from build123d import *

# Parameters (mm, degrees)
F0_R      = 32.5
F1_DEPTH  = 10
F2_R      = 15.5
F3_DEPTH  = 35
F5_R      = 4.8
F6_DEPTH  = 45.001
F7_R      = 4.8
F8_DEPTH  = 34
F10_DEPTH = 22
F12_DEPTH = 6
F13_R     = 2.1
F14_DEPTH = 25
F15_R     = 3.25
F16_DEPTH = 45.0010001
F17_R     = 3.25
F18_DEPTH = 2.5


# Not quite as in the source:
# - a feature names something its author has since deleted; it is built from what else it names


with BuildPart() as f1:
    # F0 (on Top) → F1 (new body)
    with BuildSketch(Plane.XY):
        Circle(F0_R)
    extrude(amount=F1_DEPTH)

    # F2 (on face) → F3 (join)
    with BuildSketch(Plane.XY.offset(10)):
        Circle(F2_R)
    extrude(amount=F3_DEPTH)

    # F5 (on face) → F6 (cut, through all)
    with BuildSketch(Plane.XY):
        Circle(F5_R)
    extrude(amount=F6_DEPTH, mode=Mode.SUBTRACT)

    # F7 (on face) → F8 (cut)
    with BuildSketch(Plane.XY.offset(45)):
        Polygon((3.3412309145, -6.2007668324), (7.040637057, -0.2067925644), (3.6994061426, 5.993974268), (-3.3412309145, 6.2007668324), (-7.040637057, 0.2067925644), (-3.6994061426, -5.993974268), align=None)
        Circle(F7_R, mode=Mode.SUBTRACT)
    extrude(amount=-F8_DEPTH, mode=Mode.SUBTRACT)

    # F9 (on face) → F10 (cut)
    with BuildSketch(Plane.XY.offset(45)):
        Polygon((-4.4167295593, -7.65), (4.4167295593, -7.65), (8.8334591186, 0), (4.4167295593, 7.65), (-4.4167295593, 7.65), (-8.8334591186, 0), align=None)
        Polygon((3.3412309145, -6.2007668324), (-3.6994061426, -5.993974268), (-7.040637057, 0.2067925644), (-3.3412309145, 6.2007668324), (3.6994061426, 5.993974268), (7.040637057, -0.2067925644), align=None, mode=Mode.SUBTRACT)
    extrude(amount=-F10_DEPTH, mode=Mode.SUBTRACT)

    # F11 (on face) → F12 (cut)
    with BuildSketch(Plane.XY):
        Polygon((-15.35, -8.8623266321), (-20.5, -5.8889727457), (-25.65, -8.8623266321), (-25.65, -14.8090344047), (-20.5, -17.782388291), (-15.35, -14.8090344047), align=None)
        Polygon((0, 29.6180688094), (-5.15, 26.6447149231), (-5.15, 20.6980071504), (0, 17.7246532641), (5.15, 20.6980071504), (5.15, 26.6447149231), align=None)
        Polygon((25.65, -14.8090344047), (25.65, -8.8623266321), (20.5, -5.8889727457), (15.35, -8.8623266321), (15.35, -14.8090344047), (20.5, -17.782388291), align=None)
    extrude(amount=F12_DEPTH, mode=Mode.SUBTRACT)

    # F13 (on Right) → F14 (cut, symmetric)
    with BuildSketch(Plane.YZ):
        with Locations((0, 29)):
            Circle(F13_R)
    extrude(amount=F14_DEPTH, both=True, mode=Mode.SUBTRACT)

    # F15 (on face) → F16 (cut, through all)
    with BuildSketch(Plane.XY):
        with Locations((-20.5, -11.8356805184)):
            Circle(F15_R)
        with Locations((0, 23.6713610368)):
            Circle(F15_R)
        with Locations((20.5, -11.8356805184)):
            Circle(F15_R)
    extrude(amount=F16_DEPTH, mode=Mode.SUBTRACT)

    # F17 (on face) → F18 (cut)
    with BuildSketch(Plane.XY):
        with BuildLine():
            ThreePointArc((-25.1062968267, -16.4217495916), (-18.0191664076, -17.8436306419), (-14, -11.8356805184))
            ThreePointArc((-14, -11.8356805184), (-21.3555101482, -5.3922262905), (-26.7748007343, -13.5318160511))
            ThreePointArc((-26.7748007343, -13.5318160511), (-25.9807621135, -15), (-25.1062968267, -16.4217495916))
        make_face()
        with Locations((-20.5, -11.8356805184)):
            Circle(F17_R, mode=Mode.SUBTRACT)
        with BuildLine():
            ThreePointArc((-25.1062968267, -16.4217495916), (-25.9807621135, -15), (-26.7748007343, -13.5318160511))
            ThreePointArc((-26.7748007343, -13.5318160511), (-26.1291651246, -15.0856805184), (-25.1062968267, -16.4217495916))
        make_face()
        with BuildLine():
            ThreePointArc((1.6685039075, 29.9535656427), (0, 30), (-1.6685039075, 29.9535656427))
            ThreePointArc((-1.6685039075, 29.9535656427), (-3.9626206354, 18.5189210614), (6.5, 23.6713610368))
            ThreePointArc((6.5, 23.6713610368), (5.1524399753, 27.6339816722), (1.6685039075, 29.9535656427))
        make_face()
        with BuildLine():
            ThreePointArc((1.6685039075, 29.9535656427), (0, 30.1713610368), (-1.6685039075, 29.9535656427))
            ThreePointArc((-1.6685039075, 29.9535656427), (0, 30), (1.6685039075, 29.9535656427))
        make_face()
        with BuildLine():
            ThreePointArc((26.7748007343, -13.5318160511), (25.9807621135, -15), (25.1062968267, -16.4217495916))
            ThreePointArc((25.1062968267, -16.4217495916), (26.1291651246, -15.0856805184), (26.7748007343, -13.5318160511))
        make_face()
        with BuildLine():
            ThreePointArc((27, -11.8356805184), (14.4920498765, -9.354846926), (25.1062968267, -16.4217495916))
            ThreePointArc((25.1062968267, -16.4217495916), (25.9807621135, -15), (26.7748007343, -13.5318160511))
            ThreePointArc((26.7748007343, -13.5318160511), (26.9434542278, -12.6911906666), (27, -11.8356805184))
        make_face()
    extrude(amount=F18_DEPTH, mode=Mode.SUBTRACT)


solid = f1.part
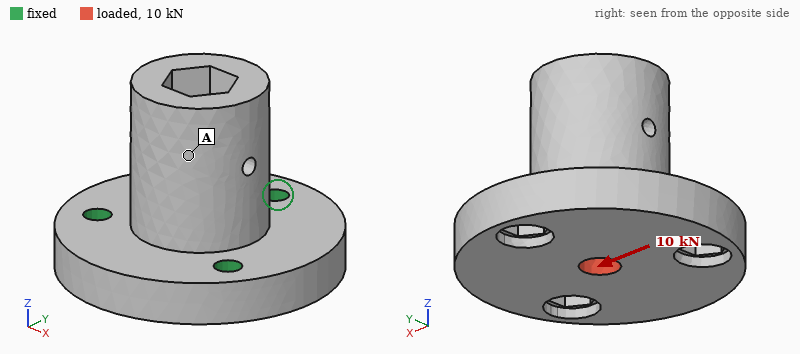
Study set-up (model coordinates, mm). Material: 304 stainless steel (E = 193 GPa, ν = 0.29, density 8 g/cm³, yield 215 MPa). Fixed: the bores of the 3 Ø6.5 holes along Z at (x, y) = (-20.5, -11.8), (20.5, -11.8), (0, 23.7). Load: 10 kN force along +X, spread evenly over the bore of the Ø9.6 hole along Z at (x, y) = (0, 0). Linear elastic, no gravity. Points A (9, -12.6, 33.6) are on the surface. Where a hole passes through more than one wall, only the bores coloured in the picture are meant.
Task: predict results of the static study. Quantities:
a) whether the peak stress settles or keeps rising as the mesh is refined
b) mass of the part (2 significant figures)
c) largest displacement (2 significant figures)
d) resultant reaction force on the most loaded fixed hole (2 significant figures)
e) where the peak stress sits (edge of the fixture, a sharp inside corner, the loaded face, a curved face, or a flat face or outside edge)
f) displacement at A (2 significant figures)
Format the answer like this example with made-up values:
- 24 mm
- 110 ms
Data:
- keeps rising
- 400 g
- 4.4 µm
- 3.6 kN
- edge of the fixture
- 1.6 µm
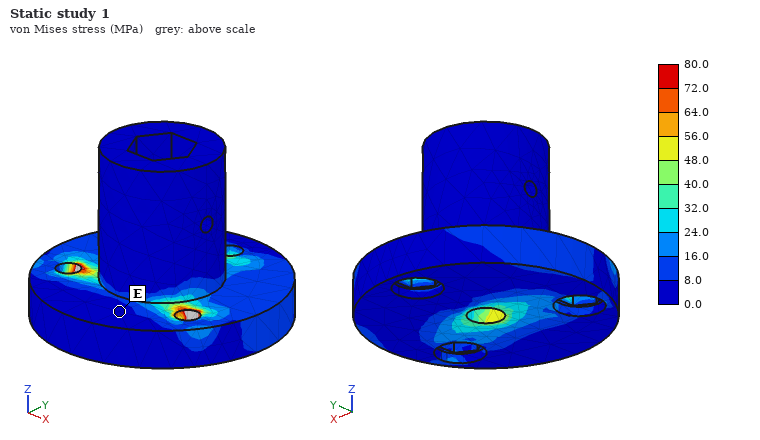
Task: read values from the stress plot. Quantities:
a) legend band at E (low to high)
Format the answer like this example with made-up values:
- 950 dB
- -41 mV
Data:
- 0.0 to 8.0 MPa
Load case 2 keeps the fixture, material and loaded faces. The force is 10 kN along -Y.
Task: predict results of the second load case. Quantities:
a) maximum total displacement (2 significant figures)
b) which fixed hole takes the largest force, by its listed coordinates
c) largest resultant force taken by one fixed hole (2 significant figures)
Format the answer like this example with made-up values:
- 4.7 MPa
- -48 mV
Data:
- 4.8 µm
- (0, 23.7)
- 3.8 kN
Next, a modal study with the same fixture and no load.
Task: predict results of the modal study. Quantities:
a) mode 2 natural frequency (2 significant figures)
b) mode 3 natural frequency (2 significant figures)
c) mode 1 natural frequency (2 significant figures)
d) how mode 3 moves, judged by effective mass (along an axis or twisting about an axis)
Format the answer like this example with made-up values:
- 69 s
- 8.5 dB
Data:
- 7100 Hz
- 11 kHz
- 7100 Hz
- along Z
